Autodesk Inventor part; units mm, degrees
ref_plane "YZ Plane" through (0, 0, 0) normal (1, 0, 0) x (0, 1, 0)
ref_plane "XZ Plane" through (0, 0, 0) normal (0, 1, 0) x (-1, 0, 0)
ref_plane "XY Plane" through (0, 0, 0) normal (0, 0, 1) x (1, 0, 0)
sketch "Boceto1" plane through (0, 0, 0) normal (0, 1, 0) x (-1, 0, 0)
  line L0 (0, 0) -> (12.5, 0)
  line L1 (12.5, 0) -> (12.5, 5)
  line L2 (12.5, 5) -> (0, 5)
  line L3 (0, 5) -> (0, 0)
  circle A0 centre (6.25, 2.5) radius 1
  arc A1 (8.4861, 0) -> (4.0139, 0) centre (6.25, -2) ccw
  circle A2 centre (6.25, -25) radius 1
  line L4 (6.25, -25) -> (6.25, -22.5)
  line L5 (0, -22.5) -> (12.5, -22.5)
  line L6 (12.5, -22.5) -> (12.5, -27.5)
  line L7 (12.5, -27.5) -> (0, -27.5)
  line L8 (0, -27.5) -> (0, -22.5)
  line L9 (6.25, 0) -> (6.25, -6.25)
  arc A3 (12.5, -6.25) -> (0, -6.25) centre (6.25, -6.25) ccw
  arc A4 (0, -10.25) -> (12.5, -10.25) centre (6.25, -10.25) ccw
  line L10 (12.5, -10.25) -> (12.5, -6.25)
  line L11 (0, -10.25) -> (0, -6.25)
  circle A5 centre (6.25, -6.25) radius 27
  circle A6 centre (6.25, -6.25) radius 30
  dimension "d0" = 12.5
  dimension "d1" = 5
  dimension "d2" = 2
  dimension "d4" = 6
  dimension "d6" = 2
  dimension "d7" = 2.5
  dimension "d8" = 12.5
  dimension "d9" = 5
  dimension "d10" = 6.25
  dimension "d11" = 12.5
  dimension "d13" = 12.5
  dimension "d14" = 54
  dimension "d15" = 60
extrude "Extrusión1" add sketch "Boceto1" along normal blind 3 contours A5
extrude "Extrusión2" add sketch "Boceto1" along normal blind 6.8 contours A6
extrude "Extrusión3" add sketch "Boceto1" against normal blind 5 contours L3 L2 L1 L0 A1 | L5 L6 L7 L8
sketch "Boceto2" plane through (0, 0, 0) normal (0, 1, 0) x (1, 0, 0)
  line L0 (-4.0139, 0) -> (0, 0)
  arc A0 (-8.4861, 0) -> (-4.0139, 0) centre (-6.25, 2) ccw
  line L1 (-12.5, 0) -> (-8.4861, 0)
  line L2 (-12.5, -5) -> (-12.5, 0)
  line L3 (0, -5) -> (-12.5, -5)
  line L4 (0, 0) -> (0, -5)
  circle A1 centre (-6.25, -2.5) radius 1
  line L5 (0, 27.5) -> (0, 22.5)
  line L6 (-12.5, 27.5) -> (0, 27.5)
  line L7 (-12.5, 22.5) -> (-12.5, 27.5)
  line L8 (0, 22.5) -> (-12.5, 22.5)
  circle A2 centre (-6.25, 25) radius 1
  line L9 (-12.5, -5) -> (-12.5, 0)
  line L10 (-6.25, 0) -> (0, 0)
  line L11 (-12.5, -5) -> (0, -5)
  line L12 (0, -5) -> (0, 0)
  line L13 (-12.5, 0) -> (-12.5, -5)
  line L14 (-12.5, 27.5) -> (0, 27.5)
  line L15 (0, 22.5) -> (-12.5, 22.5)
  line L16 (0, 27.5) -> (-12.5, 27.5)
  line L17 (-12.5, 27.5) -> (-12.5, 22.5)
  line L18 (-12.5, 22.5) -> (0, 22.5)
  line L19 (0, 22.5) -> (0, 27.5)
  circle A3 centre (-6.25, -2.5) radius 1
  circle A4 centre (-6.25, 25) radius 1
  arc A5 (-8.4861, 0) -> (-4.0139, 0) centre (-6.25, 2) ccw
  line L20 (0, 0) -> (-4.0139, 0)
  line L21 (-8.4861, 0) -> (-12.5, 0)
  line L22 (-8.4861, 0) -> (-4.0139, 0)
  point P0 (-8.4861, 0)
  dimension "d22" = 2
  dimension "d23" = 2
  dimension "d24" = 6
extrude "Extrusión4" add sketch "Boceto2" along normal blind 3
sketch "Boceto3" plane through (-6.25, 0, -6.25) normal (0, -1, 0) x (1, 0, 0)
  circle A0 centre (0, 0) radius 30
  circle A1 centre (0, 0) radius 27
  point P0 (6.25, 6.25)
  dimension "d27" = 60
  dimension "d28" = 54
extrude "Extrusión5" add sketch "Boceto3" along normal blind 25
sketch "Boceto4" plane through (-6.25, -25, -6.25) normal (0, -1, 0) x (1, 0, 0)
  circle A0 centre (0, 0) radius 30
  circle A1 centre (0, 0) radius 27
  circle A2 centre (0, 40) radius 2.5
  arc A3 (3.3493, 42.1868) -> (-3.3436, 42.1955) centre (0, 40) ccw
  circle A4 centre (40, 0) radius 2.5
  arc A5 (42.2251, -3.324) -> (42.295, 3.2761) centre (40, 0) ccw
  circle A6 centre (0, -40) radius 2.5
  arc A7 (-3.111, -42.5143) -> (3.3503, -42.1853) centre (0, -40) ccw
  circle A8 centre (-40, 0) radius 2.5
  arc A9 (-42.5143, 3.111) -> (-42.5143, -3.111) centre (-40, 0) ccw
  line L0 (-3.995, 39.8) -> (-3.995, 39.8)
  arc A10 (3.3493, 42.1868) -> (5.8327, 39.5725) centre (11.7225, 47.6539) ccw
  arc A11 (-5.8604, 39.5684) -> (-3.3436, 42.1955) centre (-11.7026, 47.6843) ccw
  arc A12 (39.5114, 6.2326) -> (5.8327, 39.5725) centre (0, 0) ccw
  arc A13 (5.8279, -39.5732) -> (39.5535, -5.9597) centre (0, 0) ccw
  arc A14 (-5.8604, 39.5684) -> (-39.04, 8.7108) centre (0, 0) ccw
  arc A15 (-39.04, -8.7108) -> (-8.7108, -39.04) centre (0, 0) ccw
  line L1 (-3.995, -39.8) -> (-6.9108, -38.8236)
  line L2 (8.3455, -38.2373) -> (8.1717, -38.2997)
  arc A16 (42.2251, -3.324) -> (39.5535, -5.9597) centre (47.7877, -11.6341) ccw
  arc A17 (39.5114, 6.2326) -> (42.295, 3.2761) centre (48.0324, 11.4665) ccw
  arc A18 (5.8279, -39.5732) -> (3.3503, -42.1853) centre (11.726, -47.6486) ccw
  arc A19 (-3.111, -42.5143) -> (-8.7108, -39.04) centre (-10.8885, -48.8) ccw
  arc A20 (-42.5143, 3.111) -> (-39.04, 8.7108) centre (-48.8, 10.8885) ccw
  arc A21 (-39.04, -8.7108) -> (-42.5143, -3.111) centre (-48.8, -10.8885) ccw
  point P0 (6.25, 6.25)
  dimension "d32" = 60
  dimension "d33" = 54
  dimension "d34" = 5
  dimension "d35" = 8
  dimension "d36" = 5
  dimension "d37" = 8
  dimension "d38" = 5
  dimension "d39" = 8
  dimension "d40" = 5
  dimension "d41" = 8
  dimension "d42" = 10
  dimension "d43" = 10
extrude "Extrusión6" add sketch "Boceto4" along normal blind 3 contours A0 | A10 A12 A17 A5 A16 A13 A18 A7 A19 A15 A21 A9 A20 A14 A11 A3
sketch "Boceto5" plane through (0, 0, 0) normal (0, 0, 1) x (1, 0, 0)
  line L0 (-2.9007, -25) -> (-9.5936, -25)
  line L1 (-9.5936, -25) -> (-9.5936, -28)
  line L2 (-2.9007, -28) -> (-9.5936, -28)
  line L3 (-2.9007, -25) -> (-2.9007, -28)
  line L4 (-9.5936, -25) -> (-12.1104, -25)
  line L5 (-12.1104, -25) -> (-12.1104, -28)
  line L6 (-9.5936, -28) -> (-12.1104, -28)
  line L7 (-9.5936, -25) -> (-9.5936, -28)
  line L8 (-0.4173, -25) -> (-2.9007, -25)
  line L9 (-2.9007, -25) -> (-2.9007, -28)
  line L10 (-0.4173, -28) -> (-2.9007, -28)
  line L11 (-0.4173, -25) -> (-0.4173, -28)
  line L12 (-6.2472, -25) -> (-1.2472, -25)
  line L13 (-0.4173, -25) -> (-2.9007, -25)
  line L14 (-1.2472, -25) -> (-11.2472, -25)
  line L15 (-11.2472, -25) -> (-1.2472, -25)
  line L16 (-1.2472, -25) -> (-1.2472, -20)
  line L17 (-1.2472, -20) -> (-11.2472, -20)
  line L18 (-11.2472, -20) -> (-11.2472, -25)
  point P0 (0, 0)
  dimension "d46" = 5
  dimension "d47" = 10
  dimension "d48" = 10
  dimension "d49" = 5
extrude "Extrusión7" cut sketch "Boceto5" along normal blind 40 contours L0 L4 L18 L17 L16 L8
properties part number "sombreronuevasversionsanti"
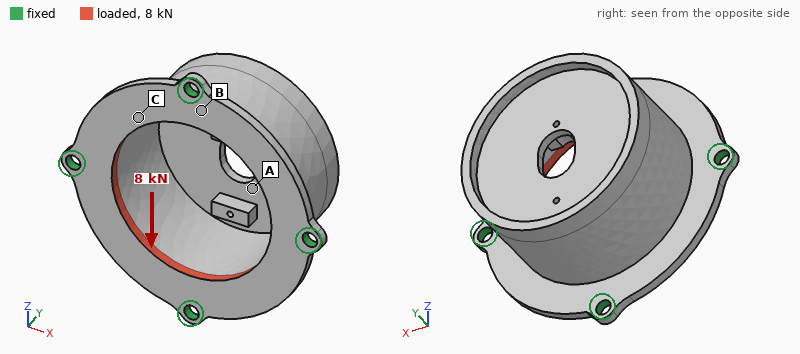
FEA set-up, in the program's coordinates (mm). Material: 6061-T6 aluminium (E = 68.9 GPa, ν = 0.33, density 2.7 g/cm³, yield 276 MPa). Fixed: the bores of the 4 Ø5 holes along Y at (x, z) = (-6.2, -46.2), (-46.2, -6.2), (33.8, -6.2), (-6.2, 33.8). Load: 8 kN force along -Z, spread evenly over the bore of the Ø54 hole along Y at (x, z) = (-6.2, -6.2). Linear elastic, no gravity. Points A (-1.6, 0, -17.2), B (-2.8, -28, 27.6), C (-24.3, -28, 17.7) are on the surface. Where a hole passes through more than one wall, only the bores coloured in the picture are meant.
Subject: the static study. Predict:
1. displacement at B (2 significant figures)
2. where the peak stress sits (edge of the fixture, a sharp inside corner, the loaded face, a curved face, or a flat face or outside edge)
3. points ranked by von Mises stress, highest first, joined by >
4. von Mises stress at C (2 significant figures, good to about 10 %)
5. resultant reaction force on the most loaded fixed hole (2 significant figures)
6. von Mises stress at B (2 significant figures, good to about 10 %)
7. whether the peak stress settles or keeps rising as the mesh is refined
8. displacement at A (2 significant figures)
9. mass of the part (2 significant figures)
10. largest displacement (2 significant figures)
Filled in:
4.4 µm
edge of the fixture
B > C > A
25 MPa
2.3 kN
48 MPa
keeps rising
14 µm
87 g
28 µm
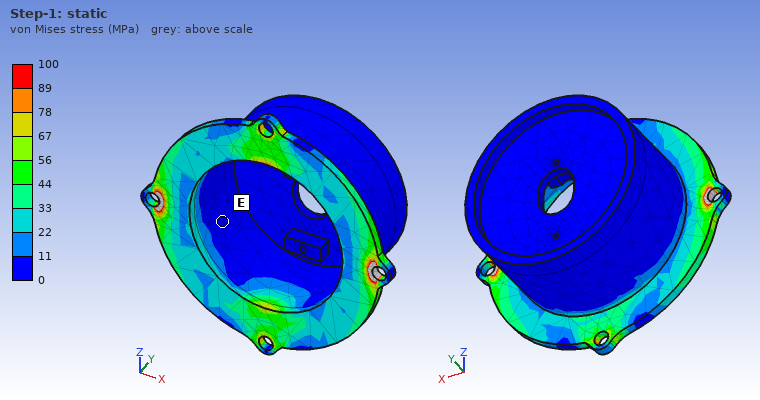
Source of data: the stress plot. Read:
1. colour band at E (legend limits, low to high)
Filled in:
0 to 11 MPa
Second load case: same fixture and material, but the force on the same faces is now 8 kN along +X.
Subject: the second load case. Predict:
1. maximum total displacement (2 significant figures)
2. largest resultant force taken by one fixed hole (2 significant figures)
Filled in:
28 µm
2.2 kN
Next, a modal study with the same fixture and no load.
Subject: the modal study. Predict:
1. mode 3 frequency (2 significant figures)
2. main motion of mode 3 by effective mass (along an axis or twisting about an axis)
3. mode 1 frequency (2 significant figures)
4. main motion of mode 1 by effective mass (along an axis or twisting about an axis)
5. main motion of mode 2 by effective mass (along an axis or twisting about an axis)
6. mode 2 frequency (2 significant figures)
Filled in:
4400 Hz
along Y
3600 Hz
along Z
along X
3900 Hz
